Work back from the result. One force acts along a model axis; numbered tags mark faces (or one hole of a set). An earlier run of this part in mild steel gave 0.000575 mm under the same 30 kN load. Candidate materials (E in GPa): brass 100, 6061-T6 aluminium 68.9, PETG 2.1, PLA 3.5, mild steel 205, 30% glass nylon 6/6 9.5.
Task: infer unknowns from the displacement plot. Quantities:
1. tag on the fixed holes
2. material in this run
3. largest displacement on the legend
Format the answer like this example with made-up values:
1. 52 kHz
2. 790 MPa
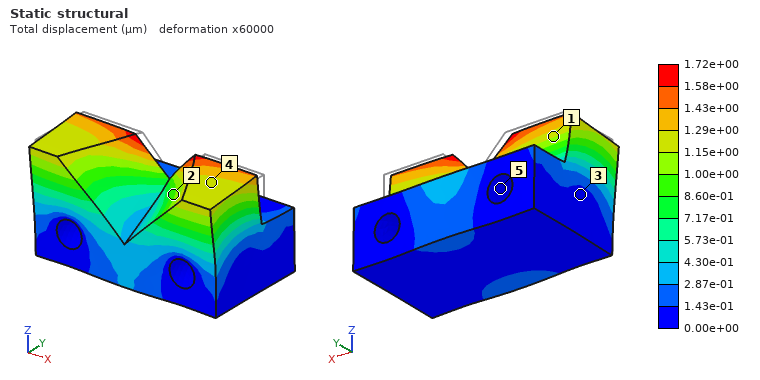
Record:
1. 5
2. 6061-T6 aluminium
3. 1.72e+00 µm
